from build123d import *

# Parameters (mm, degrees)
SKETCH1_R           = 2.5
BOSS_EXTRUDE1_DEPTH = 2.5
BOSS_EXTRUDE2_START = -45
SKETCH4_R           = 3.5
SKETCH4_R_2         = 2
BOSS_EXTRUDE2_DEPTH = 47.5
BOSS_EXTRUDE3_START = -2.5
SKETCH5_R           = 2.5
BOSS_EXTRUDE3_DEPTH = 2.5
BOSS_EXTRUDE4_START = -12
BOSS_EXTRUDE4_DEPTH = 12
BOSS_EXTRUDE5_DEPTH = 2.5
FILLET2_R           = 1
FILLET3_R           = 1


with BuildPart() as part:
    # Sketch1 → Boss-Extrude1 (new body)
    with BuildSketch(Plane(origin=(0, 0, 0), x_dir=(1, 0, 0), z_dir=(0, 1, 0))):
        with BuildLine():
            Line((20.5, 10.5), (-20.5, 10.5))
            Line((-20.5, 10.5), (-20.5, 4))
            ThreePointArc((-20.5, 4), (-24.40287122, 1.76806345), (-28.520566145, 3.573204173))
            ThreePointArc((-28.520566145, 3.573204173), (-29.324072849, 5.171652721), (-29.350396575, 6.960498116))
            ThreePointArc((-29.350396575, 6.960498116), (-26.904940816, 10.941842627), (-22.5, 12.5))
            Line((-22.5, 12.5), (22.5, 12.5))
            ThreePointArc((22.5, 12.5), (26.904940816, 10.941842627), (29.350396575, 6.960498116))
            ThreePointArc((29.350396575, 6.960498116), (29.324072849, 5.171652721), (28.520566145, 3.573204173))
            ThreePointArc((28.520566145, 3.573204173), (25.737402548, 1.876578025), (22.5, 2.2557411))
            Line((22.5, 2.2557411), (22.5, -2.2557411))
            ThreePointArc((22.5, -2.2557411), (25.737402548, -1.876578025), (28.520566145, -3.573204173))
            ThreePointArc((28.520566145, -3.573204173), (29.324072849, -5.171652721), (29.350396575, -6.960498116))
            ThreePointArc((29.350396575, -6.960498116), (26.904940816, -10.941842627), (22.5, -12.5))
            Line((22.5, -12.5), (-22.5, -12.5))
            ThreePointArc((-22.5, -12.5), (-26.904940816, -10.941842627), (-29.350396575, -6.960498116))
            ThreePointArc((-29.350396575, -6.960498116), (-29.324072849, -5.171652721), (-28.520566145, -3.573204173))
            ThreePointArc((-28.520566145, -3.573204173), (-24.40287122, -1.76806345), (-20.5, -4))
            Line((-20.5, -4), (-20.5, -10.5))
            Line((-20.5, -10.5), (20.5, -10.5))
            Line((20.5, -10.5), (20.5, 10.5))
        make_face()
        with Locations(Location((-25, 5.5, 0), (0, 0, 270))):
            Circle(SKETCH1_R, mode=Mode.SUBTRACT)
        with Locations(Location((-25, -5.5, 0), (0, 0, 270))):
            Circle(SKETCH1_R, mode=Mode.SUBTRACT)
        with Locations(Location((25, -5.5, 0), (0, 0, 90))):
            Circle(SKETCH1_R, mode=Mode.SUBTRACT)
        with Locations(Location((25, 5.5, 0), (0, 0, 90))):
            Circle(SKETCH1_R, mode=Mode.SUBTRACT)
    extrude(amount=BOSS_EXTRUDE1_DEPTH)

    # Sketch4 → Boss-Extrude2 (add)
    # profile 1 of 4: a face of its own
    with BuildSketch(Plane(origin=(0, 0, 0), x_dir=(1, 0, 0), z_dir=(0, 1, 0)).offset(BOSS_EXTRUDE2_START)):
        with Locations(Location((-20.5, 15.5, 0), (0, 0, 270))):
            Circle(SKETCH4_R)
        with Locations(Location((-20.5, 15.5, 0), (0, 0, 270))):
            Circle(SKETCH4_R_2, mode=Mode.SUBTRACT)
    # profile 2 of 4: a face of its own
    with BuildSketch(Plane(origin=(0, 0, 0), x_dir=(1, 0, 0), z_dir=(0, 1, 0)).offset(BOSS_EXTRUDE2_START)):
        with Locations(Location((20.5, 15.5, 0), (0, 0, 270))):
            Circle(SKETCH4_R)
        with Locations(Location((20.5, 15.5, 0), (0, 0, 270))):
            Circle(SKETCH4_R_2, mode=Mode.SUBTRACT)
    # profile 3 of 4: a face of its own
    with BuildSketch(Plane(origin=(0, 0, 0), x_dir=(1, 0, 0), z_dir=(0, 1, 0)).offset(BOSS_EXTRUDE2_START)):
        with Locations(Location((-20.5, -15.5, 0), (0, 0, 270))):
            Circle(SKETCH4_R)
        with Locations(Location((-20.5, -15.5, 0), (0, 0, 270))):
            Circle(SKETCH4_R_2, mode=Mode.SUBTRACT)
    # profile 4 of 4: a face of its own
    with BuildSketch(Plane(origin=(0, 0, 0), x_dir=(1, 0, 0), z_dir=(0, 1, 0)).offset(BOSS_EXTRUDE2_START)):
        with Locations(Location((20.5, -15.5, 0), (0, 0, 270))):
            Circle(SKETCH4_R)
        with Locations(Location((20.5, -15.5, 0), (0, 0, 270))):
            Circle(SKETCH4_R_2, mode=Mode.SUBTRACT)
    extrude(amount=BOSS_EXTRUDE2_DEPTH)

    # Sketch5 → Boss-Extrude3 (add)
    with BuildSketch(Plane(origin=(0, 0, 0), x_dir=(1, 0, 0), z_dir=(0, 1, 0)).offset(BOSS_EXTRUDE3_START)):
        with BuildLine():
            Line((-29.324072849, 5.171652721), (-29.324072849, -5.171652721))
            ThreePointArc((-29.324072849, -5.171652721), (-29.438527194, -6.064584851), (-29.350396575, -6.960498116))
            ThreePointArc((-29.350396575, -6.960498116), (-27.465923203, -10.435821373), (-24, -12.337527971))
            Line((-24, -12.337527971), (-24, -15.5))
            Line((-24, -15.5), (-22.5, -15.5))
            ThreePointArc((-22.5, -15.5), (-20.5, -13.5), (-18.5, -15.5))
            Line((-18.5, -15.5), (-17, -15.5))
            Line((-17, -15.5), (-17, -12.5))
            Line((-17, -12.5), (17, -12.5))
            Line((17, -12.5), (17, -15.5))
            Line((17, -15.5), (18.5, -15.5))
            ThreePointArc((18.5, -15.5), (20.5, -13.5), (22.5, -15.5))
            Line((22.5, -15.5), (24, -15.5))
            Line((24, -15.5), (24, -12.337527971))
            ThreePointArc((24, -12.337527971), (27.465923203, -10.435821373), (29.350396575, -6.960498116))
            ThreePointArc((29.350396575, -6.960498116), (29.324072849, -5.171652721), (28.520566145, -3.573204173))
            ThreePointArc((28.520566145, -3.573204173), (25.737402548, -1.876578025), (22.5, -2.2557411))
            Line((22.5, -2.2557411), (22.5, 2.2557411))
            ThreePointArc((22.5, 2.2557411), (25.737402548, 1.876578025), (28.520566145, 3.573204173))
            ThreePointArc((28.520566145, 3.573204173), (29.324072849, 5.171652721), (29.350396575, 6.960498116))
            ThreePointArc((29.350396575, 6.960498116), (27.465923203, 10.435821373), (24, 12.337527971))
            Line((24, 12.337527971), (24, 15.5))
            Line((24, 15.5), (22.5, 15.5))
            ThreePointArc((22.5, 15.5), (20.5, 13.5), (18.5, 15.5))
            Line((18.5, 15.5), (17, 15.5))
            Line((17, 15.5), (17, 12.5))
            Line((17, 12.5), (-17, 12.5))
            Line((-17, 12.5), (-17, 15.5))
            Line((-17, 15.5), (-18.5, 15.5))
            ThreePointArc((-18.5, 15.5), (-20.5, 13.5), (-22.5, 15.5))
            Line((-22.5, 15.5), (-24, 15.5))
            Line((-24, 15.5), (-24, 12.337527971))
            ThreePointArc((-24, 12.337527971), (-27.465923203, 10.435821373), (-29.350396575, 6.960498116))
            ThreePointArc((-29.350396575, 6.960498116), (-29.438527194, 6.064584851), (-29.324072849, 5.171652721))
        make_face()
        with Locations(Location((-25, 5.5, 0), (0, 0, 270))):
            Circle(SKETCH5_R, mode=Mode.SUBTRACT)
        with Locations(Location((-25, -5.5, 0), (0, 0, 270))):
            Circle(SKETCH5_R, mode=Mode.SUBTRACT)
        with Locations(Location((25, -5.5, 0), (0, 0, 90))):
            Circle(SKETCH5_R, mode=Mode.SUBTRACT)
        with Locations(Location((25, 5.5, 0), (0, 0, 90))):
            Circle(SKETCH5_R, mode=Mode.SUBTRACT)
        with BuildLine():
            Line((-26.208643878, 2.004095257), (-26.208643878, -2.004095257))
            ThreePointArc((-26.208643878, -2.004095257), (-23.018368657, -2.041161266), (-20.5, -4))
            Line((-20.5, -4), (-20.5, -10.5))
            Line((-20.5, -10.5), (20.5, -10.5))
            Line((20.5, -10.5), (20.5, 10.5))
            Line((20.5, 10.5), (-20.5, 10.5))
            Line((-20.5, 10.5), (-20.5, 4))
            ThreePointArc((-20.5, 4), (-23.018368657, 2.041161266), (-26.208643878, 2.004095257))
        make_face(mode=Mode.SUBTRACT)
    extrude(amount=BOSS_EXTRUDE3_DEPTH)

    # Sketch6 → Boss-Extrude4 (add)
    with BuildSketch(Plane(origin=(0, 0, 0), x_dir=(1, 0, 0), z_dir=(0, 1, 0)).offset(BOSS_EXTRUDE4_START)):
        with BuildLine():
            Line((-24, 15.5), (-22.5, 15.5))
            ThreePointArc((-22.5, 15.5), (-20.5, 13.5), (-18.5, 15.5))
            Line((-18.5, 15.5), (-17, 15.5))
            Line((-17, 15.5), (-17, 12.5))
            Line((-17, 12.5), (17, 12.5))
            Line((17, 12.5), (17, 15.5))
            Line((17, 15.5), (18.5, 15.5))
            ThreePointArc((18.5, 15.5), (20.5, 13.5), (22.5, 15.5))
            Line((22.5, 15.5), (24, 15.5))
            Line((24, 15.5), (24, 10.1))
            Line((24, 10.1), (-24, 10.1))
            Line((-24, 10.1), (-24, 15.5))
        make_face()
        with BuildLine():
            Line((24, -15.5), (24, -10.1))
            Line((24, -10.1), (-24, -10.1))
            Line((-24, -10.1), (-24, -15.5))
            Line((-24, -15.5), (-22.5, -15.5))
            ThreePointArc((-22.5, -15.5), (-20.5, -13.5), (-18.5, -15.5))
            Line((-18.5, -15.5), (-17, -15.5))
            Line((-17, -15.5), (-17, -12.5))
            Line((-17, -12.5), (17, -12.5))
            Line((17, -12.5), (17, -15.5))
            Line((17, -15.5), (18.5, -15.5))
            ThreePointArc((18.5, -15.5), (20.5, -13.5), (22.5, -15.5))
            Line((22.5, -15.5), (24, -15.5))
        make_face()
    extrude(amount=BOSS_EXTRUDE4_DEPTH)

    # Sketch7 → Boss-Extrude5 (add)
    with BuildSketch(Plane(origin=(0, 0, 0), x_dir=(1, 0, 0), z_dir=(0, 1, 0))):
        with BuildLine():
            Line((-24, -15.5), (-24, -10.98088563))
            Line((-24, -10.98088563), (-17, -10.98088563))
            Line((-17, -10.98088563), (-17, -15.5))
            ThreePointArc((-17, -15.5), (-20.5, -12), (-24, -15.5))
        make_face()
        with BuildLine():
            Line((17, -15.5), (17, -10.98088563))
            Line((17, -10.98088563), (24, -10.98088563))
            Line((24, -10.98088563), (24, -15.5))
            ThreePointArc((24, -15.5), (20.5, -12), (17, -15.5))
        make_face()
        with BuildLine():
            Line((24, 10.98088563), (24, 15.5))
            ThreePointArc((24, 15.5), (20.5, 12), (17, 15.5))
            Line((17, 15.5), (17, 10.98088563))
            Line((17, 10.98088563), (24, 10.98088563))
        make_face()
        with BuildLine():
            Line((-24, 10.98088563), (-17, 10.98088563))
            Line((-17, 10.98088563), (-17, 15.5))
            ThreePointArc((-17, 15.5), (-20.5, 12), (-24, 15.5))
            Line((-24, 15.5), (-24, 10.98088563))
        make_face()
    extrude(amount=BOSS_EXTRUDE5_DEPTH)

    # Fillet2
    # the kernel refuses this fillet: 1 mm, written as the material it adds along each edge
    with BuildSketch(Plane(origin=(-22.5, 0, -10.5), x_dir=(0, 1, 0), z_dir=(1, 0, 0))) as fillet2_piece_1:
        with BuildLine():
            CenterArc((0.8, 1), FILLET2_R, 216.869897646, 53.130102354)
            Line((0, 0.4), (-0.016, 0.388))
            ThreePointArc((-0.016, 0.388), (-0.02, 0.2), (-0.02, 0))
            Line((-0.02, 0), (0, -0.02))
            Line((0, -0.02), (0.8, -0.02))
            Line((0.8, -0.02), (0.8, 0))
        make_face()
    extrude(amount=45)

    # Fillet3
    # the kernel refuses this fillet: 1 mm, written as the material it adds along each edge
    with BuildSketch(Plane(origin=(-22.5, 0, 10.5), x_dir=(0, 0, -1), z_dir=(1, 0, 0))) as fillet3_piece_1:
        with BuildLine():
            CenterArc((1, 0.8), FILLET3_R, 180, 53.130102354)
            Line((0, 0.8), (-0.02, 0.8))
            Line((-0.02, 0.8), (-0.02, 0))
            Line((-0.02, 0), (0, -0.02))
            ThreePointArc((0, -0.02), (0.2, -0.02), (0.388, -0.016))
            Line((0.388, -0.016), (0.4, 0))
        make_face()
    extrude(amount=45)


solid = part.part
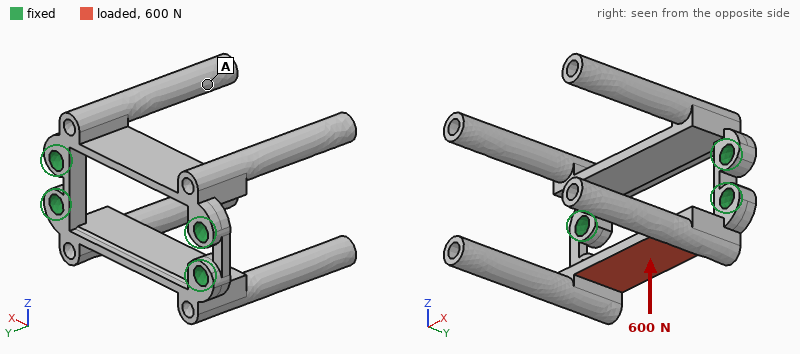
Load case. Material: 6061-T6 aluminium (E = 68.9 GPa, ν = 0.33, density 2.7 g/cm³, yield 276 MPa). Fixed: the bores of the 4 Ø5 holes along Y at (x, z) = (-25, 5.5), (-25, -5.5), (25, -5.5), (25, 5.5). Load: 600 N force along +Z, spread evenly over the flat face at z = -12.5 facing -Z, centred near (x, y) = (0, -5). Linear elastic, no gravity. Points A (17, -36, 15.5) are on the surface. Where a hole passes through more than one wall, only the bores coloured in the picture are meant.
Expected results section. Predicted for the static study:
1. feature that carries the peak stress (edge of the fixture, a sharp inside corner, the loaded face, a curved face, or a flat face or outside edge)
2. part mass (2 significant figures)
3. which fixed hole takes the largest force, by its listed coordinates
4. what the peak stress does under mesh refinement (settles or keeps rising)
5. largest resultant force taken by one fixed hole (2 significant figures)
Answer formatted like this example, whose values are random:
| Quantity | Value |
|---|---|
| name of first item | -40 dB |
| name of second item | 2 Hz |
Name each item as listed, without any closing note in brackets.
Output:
| Quantity | Value |
|---|---|
| feature that carries the peak stress | a sharp inside corner |
| part mass | 25 g |
| which fixed hole takes the largest force, by its listed coordinates | (-25, -5.5) |
| what the peak stress does under mesh refinement | keeps rising |
| largest resultant force taken by one fixed hole | 340 N |
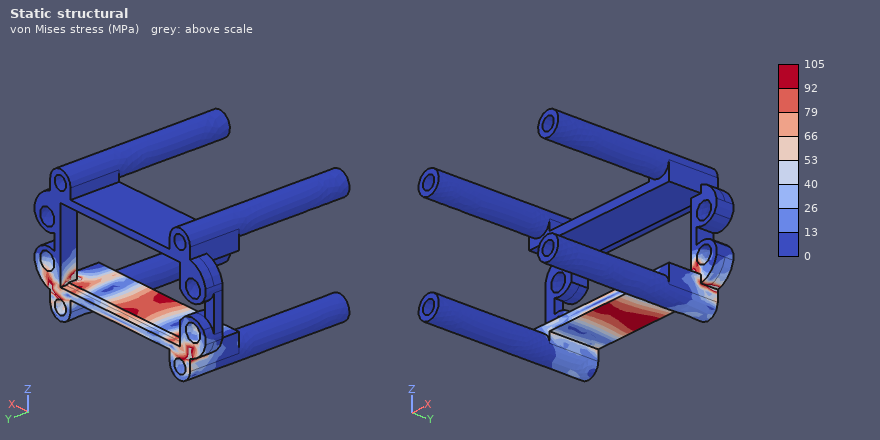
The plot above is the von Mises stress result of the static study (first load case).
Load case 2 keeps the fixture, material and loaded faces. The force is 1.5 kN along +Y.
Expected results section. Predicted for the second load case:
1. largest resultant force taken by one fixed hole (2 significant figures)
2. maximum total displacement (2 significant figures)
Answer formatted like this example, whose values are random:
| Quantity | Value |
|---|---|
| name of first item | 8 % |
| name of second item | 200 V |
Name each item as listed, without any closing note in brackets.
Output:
| Quantity | Value |
|---|---|
| largest resultant force taken by one fixed hole | 930 N |
| maximum total displacement | 0.16 mm |
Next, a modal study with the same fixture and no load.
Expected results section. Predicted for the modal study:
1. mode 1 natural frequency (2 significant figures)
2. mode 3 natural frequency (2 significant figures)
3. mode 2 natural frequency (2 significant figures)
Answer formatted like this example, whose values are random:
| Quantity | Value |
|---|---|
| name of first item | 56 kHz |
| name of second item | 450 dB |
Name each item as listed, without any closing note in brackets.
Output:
| Quantity | Value |
|---|---|
| mode 1 natural frequency | 2200 Hz |
| mode 3 natural frequency | 2300 Hz |
| mode 2 natural frequency | 2200 Hz |
